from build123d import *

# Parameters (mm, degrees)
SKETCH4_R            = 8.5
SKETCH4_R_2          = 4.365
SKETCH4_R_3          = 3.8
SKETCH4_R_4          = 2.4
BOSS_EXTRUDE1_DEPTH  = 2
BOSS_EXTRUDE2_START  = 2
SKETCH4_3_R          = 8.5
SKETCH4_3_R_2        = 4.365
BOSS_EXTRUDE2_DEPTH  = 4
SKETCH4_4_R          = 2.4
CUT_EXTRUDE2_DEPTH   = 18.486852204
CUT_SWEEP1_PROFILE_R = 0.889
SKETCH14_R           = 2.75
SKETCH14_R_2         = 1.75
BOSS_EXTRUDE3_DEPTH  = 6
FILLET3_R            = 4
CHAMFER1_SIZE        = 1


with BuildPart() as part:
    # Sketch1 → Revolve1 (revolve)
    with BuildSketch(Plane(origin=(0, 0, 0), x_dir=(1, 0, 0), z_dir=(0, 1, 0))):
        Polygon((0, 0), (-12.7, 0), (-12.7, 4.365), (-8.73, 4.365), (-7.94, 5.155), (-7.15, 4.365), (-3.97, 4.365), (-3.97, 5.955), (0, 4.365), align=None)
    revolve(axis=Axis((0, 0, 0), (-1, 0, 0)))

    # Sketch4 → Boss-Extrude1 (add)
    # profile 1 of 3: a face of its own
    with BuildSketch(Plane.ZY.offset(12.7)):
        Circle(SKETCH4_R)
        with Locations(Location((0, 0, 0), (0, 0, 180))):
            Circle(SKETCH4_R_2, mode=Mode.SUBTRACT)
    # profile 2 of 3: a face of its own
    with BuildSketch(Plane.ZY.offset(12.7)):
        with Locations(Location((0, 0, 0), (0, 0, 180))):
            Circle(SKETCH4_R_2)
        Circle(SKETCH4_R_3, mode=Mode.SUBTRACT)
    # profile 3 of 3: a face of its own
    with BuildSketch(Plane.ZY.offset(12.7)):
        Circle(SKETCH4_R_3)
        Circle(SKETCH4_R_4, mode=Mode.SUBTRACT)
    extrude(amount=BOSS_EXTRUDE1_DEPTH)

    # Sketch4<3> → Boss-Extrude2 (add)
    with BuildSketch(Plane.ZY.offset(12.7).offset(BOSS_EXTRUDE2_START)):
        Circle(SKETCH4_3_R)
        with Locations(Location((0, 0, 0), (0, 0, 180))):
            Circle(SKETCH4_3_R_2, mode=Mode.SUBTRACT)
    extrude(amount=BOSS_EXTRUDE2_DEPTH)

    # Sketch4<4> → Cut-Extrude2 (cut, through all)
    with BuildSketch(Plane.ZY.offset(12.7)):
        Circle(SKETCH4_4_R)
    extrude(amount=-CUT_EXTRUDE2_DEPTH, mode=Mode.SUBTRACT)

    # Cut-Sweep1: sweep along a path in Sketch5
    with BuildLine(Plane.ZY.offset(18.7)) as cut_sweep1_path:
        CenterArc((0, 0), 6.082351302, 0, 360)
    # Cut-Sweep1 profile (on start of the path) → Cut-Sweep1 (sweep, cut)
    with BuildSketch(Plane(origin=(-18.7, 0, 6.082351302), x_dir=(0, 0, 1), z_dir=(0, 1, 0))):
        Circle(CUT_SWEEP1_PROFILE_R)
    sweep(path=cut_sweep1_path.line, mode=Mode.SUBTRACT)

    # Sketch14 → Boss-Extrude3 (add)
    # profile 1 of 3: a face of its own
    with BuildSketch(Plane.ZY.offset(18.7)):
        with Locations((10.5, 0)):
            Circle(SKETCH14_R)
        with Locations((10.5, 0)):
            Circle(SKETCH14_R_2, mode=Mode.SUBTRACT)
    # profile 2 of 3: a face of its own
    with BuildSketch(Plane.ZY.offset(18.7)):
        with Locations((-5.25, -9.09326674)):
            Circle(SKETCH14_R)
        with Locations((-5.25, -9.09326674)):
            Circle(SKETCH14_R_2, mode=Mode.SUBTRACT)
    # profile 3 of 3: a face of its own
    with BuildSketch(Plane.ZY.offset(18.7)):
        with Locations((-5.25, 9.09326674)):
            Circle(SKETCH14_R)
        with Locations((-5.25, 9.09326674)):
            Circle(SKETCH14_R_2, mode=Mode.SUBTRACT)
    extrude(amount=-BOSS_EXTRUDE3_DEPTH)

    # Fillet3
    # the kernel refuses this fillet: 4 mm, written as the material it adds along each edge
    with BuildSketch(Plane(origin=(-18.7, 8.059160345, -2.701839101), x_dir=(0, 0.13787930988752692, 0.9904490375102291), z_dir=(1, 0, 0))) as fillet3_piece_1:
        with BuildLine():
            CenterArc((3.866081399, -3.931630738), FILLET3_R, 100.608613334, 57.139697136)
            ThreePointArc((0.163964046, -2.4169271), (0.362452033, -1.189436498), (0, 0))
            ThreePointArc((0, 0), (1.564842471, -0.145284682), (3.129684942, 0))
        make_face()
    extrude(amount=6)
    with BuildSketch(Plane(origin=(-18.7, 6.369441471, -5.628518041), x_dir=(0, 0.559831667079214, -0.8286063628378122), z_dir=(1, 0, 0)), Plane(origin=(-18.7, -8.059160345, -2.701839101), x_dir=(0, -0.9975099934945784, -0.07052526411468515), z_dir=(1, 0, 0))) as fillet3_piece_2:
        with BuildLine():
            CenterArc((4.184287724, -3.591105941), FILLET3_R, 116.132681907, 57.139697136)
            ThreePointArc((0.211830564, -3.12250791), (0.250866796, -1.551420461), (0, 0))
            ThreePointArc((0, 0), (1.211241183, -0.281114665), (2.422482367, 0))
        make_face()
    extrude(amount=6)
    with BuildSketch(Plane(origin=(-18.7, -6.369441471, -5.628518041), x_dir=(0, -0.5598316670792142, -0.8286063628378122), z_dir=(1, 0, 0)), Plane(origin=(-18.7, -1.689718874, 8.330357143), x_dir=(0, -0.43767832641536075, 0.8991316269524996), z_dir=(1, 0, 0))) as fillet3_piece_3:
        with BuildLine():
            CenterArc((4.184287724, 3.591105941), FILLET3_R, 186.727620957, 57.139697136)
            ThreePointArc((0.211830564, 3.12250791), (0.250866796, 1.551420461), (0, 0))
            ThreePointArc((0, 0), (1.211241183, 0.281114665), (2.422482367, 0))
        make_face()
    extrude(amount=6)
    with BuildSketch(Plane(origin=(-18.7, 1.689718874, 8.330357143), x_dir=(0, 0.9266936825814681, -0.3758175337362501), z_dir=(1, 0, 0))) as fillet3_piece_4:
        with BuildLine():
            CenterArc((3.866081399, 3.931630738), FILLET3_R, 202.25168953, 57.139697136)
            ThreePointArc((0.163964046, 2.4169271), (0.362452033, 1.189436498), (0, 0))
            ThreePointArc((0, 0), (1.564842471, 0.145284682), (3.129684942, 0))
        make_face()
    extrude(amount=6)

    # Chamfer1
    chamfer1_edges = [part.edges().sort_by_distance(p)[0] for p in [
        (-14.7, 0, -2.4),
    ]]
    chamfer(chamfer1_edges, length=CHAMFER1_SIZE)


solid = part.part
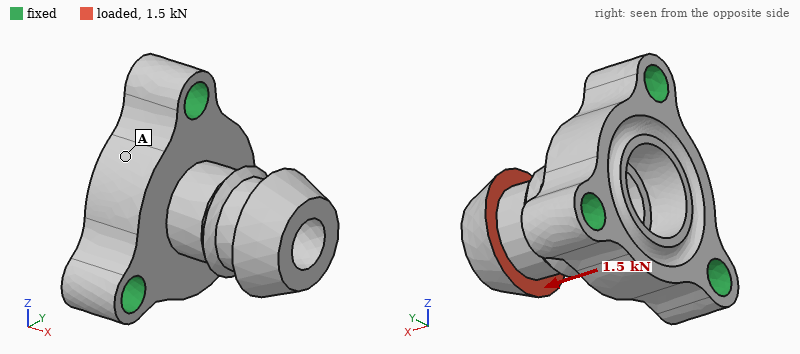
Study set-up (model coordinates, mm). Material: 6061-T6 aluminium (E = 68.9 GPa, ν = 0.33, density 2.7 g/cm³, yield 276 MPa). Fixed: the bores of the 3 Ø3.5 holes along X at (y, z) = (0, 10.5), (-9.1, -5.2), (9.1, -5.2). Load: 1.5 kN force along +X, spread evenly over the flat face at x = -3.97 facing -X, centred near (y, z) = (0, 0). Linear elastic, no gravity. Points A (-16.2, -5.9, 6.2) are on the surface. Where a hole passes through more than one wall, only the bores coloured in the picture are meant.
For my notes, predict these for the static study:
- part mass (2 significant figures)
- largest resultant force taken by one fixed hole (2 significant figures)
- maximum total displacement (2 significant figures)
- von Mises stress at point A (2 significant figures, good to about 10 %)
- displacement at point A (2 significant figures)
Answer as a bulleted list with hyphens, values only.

- 5.3 g
- 540 N
- 14 µm
- 9.9 MPa
- 2.6 µm
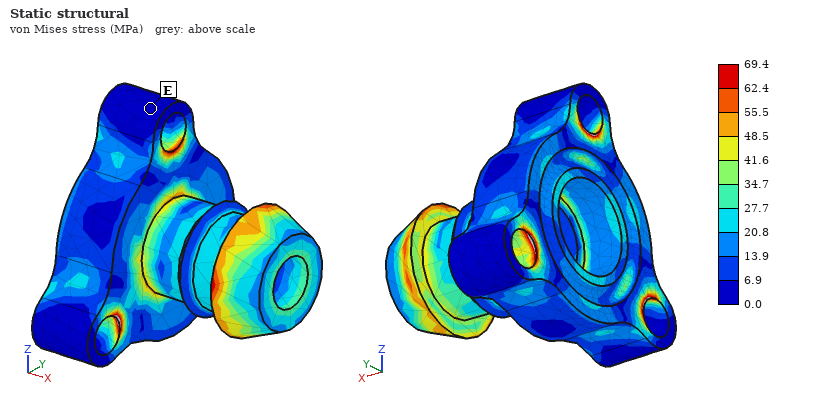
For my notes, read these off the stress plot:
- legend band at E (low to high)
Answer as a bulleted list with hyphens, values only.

- 0.0 to 6.9 MPa
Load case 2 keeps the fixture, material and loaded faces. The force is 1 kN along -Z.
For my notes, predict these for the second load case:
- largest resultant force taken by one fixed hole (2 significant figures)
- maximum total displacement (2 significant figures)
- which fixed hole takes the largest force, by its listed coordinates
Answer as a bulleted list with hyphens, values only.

- 1.0 kN
- 69 µm
- (0, 10.5)
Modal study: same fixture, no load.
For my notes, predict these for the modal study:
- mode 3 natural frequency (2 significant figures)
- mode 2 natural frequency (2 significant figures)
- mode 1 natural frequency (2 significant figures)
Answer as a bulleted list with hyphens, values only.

- 44 kHz
- 19 kHz
- 19 kHz
